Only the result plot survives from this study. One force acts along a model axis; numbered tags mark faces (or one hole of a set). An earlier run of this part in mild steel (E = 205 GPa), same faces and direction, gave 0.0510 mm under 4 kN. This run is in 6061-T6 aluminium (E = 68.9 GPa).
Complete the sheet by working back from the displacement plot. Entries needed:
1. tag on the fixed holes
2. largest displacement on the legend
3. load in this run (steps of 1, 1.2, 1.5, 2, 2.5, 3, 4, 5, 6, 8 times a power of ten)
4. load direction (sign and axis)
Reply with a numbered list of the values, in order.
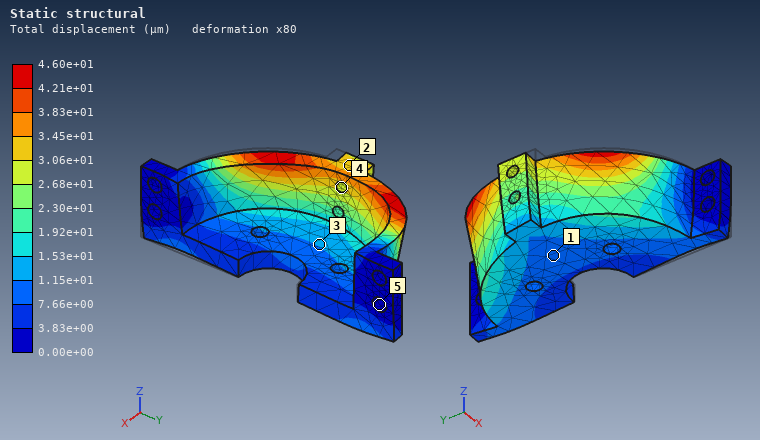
1. 5
2. 4.60e+01 µm
3. 1.2 kN
4. +Y
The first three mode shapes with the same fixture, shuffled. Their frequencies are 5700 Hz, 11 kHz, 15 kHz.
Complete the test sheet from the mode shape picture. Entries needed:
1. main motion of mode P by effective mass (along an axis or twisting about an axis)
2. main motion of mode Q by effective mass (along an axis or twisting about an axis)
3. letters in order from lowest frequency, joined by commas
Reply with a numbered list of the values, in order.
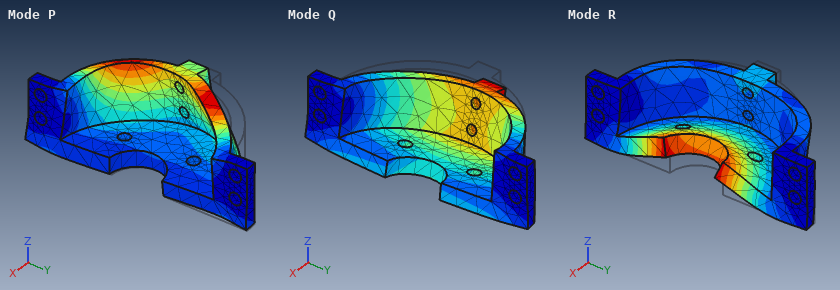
1. along Y
2. along Z
3. Q, P, R
